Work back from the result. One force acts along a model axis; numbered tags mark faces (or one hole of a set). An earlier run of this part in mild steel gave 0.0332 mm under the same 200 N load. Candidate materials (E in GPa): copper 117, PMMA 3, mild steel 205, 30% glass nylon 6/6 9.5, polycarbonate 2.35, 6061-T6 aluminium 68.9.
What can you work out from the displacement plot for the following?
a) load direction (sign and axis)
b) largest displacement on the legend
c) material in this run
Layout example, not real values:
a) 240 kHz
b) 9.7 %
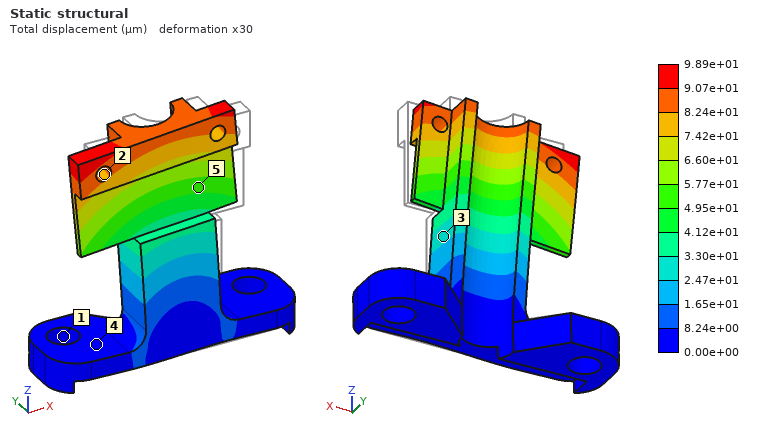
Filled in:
a) -X
b) 9.89e+01 µm
c) 6061-T6 aluminium
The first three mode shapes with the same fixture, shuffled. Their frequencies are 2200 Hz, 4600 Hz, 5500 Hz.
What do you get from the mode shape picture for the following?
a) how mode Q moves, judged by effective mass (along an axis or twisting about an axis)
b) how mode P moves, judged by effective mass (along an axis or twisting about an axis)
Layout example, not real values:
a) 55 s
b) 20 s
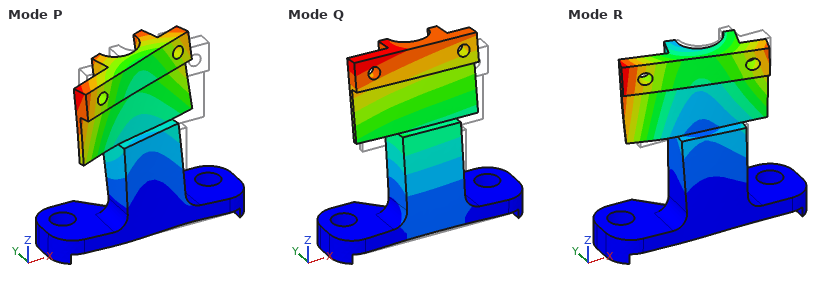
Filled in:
a) along Y
b) along X
